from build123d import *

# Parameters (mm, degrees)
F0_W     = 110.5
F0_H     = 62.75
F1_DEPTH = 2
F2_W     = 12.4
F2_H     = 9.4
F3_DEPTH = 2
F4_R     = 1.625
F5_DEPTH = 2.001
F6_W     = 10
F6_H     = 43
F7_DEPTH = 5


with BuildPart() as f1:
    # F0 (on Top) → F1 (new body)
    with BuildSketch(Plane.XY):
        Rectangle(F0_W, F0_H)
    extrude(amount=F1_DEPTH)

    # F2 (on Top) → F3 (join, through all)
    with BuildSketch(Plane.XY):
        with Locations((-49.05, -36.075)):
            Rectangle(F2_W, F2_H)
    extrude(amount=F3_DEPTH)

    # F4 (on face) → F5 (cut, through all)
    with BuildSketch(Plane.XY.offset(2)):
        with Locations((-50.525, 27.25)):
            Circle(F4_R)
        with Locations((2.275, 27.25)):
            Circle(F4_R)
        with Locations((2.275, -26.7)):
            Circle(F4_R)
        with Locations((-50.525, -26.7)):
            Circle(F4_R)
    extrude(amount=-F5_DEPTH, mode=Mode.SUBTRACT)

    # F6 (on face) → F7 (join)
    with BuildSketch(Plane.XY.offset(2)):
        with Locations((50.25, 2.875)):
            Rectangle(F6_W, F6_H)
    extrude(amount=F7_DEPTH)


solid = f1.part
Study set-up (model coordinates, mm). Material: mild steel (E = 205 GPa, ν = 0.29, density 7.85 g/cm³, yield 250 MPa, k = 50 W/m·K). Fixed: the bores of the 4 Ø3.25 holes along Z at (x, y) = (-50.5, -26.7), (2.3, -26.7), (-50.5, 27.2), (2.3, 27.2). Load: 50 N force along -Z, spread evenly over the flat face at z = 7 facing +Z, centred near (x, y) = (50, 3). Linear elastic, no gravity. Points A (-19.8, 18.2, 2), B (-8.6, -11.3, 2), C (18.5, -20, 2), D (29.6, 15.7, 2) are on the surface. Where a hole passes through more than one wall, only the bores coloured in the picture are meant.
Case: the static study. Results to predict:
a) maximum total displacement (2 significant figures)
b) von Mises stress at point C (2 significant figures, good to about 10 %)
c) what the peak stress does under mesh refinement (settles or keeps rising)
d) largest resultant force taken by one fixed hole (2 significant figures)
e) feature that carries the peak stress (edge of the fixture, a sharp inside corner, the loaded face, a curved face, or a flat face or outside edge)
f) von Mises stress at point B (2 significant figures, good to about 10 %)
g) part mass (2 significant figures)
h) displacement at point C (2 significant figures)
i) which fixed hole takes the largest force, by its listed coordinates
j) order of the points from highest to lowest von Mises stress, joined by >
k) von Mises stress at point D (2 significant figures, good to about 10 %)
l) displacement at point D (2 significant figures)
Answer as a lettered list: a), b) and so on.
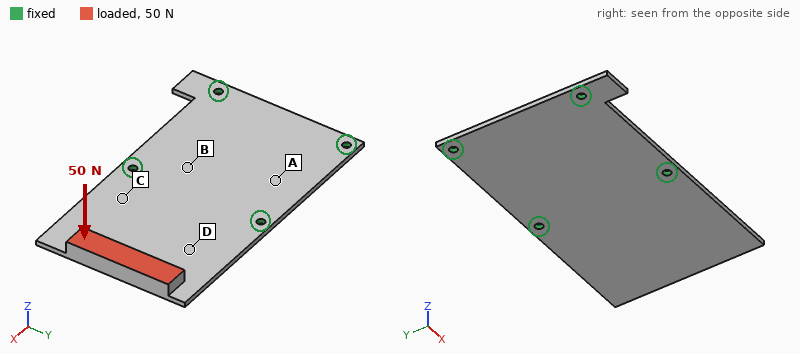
a) 0.30 mm
b) 36 MPa
c) keeps rising
d) 35 N
e) edge of the fixture
f) 13 MPa
g) 130 g
h) 0.046 mm
i) (2.3, 27.2)
j) C > D > B > A
k) 25 MPa
l) 0.11 mm
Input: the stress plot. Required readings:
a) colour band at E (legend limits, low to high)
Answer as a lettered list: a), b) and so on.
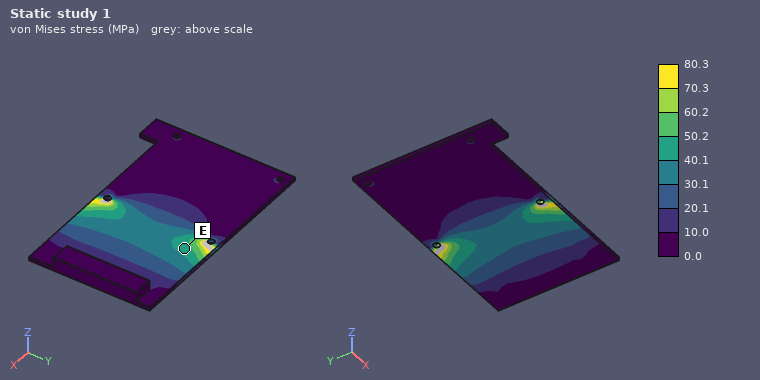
a) 40.1 to 50.2 MPa
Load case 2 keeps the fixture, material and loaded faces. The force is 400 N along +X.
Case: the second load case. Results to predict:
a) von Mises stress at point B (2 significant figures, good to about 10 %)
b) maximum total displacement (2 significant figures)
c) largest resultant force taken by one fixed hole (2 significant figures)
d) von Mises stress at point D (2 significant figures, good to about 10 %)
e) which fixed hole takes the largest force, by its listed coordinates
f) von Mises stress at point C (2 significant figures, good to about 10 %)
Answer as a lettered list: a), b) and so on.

a) 15 MPa
b) 0.42 mm
c) 180 N
d) 57 MPa
e) (2.3, 27.2)
f) 57 MPa
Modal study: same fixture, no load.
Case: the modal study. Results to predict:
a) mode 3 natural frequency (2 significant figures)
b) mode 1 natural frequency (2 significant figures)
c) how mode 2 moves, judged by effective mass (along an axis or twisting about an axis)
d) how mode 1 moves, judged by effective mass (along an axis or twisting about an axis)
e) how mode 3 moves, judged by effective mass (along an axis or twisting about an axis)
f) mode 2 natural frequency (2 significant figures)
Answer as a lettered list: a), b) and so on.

a) 2500 Hz
b) 380 Hz
c) twisting about X
d) along Z
e) along Z
f) 1300 Hz
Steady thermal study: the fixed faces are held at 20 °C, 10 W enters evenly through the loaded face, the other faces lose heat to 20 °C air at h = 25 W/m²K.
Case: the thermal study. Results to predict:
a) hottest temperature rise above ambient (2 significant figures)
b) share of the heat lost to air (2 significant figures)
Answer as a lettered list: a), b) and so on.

a) 55 K
b) 58 %
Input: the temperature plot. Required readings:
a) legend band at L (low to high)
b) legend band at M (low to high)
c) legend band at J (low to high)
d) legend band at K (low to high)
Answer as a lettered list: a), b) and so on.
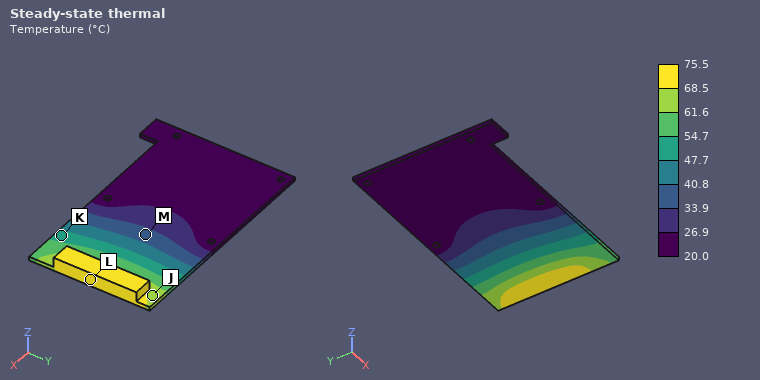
a) 68.5 to 75.5 °C
b) 33.9 to 40.8 °C
c) 61.6 to 68.5 °C
d) 47.7 to 54.7 °C
